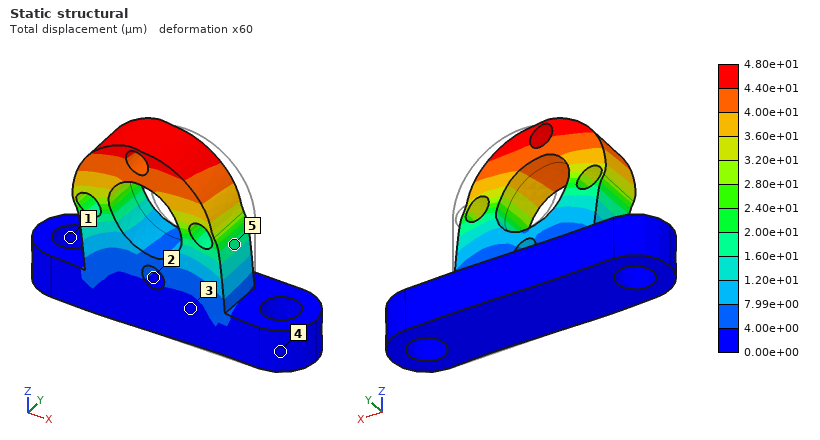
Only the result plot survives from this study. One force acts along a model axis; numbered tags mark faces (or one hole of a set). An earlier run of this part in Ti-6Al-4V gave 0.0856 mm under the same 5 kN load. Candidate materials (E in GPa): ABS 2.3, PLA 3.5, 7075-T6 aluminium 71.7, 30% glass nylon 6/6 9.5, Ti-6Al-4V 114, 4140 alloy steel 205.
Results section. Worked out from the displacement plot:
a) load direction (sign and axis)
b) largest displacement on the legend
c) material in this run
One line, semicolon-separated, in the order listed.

-X; 4.80e+01 µm; 4140 alloy steel
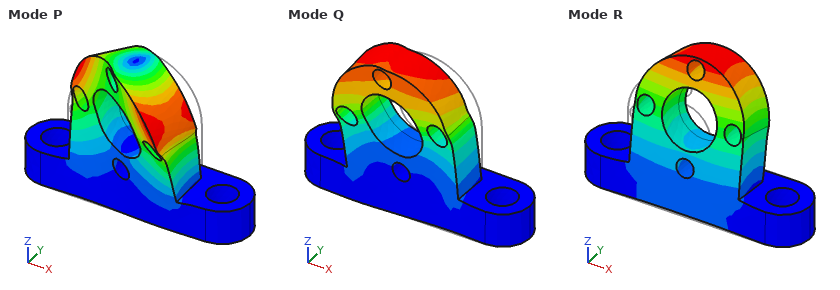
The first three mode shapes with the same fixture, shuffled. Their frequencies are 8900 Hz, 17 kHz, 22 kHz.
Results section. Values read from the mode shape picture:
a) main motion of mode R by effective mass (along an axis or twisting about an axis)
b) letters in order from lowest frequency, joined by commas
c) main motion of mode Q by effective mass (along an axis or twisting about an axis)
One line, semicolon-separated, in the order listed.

along Y; R, Q, P; along X
